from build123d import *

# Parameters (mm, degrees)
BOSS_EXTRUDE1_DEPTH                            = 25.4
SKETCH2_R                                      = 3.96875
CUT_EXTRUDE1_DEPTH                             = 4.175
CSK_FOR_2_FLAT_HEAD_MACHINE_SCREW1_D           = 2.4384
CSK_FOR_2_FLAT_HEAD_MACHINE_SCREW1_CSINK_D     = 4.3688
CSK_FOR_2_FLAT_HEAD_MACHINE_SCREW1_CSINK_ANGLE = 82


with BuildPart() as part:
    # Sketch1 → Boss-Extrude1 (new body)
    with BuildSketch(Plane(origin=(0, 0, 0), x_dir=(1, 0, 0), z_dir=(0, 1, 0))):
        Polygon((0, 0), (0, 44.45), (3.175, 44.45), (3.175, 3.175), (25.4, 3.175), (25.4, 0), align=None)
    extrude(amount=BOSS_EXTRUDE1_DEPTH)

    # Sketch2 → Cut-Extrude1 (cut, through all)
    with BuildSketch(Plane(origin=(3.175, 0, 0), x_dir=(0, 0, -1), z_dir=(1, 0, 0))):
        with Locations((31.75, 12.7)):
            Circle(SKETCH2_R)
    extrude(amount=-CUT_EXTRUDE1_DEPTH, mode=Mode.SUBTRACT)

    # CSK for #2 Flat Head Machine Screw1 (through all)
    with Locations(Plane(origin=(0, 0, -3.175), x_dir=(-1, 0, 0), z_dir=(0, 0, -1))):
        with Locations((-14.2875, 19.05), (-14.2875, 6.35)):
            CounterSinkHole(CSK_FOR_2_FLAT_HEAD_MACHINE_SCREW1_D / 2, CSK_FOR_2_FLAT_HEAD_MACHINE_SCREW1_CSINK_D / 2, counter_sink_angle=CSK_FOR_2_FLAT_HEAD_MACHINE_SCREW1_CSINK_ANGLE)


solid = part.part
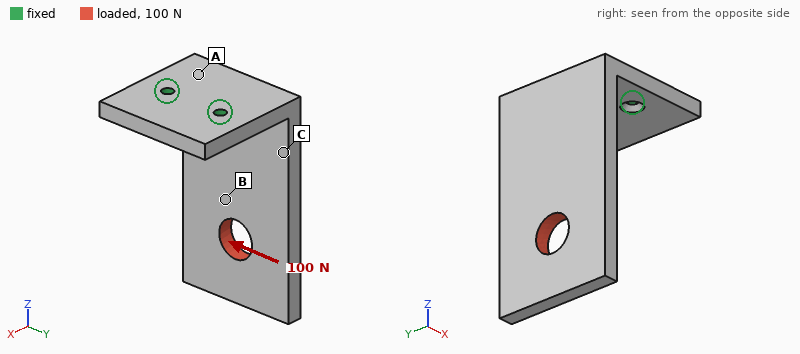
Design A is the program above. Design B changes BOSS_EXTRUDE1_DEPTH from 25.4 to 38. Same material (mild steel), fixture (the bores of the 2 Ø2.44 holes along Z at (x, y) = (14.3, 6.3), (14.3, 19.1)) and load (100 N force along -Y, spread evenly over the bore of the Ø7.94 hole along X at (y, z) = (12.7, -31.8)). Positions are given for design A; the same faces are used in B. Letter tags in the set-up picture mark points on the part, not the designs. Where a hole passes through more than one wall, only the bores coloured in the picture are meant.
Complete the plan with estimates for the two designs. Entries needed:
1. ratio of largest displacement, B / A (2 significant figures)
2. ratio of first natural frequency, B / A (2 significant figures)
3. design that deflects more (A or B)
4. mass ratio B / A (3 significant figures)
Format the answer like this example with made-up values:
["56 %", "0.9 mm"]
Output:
["0.89", "0.92", "A", "1.51"]
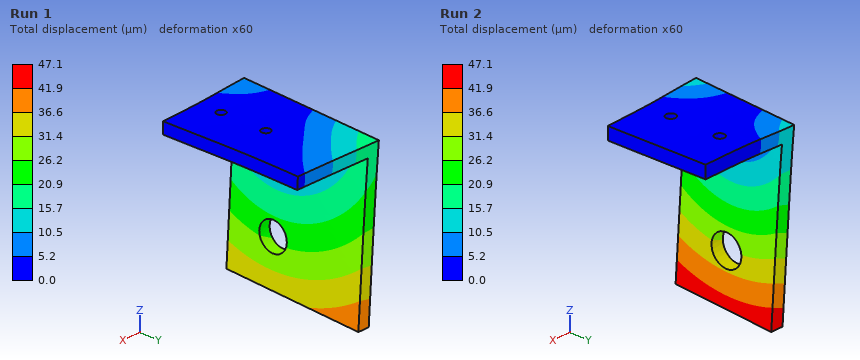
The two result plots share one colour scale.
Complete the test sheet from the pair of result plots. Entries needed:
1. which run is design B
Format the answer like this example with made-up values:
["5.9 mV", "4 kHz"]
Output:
["Run 1"]
